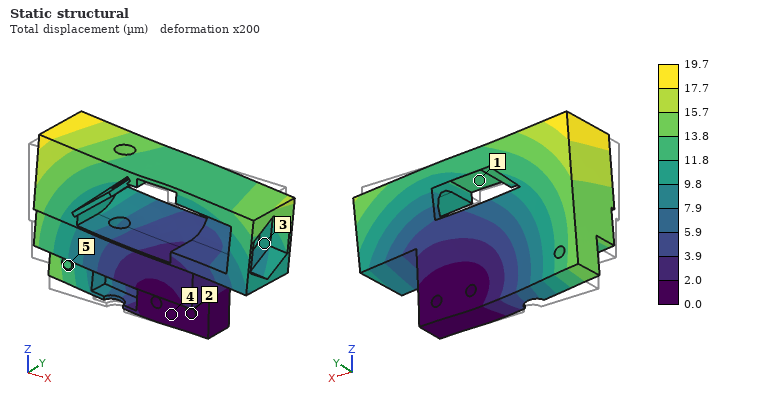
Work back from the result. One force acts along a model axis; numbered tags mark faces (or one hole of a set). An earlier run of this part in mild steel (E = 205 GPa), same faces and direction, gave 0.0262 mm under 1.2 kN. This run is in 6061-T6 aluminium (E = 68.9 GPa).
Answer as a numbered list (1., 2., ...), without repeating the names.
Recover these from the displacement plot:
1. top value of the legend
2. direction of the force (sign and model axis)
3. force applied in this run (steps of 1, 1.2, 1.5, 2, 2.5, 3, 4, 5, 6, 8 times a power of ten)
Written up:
1. 19.7 µm
2. +Z
3. 300 N
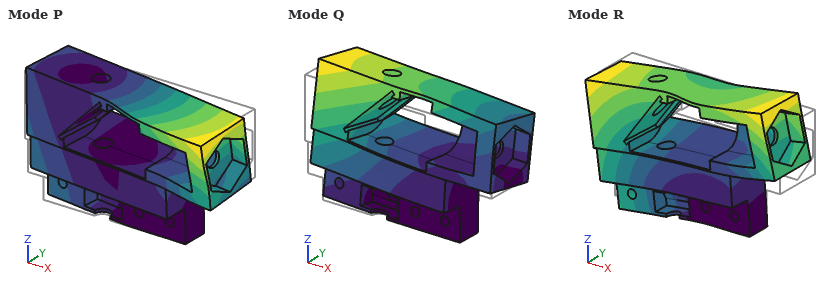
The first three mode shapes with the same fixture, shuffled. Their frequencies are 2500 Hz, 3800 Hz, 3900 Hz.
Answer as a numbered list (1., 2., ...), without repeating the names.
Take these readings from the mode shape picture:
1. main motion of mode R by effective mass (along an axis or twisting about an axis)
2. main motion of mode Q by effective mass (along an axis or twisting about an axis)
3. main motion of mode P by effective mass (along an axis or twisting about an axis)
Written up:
1. along X
2. along Y
3. twisting about Z
